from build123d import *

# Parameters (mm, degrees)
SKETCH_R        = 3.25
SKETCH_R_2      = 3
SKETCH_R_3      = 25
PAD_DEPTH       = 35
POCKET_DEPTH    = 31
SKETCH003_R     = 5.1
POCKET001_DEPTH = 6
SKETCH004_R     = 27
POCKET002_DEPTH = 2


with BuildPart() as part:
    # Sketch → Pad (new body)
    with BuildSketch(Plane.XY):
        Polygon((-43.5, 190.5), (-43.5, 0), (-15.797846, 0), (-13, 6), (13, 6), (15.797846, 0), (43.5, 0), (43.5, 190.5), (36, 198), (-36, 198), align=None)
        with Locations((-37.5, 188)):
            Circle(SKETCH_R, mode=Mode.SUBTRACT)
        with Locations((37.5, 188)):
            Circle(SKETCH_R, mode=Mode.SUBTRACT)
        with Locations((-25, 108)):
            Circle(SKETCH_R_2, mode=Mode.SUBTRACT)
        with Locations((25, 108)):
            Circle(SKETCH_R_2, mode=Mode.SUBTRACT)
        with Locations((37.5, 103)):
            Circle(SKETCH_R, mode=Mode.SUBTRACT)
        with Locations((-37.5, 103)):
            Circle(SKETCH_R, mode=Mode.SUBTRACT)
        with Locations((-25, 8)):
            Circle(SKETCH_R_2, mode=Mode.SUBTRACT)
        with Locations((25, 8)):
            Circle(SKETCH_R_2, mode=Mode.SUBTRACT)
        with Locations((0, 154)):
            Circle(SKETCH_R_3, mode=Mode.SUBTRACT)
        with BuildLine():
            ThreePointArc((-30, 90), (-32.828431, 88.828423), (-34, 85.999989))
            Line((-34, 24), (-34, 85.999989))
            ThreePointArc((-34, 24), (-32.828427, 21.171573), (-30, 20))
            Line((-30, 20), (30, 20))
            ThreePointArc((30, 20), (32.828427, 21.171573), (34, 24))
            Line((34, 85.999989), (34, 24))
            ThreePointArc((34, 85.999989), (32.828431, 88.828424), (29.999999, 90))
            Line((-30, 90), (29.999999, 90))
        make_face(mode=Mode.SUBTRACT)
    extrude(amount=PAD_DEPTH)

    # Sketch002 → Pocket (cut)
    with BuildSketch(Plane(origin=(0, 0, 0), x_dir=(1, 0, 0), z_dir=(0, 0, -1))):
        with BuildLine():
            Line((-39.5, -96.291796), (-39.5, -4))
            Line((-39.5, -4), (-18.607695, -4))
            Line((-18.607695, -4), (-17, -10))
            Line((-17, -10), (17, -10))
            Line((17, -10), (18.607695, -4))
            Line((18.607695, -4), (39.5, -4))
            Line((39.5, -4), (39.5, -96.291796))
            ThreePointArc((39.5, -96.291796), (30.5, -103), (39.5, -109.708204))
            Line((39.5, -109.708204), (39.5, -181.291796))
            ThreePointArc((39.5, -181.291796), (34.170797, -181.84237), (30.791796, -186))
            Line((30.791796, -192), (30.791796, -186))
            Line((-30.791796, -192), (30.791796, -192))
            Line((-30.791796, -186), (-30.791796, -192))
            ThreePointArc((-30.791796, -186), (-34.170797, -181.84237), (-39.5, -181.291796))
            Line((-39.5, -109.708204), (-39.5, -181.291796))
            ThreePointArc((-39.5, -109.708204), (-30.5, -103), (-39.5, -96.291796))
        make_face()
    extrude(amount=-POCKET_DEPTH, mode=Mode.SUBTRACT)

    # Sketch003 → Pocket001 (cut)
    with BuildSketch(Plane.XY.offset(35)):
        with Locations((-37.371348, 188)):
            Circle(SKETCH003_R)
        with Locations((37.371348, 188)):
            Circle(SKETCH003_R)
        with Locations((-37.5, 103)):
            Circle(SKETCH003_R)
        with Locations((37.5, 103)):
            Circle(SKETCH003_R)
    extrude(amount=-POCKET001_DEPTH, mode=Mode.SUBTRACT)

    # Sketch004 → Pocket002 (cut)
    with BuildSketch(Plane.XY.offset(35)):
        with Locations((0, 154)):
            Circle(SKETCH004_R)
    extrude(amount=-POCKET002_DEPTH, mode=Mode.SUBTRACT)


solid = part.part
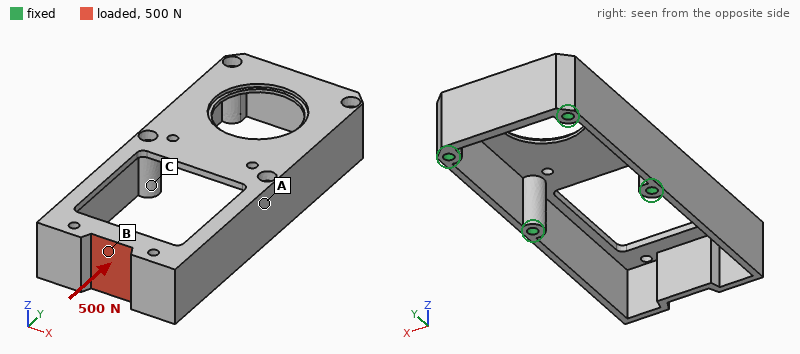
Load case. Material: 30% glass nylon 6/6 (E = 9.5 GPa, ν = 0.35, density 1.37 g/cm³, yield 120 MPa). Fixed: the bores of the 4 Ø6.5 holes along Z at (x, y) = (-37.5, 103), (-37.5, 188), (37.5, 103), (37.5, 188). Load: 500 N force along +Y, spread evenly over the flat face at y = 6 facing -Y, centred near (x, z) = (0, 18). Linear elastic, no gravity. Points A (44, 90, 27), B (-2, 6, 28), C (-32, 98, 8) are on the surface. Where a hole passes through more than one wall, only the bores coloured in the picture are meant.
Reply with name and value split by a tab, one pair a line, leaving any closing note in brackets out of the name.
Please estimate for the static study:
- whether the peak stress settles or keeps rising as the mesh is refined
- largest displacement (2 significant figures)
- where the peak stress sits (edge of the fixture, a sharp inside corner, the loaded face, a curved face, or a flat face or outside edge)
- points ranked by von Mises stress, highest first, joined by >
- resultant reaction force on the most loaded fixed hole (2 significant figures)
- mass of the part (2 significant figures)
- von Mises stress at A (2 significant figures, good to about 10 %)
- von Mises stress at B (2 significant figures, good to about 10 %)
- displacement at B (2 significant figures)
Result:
whether the peak stress settles or keeps rising as the mesh is refined	keeps rising
largest displacement	0.76 mm
where the peak stress sits	a sharp inside corner
points ranked by von Mises stress, highest first, joined by >	B > A > C
resultant reaction force on the most loaded fixed hole	250 N
mass of the part	160 g
von Mises stress at A	5.0 MPa
von Mises stress at B	20 MPa
displacement at B	0.33 mm
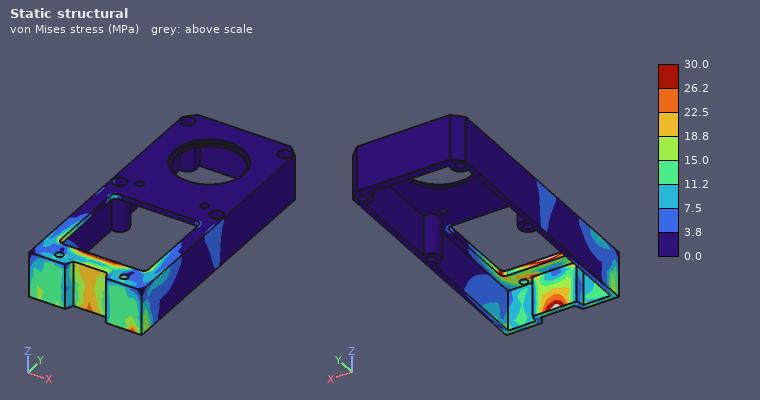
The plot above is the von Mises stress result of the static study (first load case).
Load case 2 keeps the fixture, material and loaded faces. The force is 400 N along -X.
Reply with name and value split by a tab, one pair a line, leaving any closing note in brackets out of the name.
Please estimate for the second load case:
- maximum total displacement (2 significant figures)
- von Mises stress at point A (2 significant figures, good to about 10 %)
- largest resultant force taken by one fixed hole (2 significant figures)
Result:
maximum total displacement	2.3 mm
von Mises stress at point A	37 MPa
largest resultant force taken by one fixed hole	460 N
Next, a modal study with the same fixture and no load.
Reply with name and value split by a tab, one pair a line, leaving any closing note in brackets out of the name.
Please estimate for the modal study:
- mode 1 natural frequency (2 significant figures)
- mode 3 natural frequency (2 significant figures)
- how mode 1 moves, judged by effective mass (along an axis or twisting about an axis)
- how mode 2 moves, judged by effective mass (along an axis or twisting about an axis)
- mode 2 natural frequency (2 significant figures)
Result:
mode 1 natural frequency	350 Hz
mode 3 natural frequency	1100 Hz
how mode 1 moves, judged by effective mass	along X
how mode 2 moves, judged by effective mass	along Z
mode 2 natural frequency	810 Hz
